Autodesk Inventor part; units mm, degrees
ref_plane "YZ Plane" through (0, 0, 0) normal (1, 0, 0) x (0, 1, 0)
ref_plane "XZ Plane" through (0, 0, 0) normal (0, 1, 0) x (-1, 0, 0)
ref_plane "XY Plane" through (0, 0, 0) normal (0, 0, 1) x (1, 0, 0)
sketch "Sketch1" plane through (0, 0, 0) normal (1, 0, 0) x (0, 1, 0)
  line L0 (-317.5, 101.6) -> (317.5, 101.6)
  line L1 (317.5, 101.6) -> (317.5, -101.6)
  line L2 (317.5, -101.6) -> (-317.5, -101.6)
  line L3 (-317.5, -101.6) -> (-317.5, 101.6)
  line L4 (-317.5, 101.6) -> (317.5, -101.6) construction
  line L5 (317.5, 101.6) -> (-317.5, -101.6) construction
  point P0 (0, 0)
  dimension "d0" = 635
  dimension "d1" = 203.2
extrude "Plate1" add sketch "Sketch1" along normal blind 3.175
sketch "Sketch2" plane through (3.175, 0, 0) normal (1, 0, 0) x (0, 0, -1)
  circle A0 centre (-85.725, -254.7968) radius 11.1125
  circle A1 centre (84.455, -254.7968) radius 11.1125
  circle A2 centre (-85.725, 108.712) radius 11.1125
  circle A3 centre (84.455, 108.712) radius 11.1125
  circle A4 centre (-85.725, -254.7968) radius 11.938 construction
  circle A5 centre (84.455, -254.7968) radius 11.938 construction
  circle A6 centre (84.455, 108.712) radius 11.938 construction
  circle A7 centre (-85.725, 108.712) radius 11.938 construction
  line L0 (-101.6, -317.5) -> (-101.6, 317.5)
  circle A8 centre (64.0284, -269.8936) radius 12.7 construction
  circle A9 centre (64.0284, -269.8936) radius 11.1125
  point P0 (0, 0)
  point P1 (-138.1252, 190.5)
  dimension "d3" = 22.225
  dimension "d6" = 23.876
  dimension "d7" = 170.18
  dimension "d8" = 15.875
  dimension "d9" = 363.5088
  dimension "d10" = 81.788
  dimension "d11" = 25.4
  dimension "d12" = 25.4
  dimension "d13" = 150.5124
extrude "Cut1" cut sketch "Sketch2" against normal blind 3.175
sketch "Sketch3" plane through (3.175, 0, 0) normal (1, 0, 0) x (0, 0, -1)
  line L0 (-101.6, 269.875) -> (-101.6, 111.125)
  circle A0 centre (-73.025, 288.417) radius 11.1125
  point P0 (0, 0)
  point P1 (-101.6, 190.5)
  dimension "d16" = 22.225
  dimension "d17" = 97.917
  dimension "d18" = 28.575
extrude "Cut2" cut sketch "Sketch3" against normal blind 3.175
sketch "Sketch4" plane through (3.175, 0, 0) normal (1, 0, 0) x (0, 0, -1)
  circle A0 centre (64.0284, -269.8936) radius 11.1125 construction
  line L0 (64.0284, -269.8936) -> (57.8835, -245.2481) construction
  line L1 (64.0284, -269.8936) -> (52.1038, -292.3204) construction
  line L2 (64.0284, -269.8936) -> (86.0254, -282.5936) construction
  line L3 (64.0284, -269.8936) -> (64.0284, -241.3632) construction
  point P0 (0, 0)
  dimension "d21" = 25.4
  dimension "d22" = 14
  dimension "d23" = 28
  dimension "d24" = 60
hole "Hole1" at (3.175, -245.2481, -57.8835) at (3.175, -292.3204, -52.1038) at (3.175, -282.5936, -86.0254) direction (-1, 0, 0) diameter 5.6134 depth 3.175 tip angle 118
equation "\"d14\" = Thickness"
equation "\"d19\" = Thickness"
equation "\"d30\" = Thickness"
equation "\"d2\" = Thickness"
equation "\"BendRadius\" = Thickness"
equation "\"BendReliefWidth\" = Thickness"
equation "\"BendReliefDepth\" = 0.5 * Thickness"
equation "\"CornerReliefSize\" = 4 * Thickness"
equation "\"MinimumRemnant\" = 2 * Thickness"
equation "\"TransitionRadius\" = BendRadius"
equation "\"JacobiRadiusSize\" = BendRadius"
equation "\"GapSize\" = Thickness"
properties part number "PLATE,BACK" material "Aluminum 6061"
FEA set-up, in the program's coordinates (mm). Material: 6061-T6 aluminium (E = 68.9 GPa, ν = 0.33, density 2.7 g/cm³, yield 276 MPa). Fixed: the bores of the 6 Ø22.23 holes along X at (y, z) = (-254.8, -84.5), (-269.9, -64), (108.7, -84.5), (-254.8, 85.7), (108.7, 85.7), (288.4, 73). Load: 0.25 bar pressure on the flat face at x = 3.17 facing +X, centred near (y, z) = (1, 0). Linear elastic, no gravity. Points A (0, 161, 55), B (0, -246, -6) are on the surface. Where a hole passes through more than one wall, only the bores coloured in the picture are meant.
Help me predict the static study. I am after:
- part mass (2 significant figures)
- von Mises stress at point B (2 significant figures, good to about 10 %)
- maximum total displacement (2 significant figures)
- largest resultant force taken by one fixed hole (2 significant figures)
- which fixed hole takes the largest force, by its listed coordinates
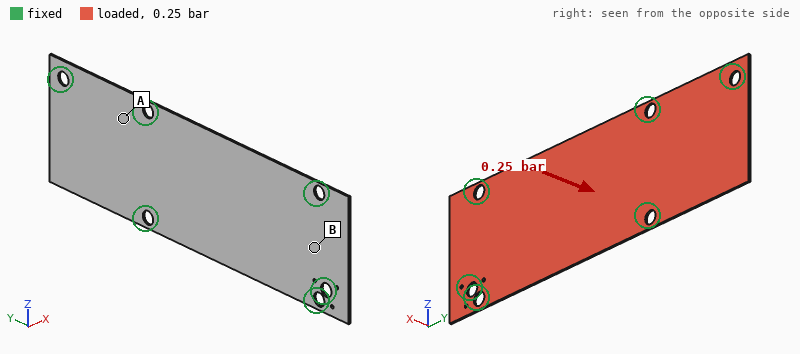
1.1 kg
60 MPa
6.0 mm
850 N
(108.7, -84.5)
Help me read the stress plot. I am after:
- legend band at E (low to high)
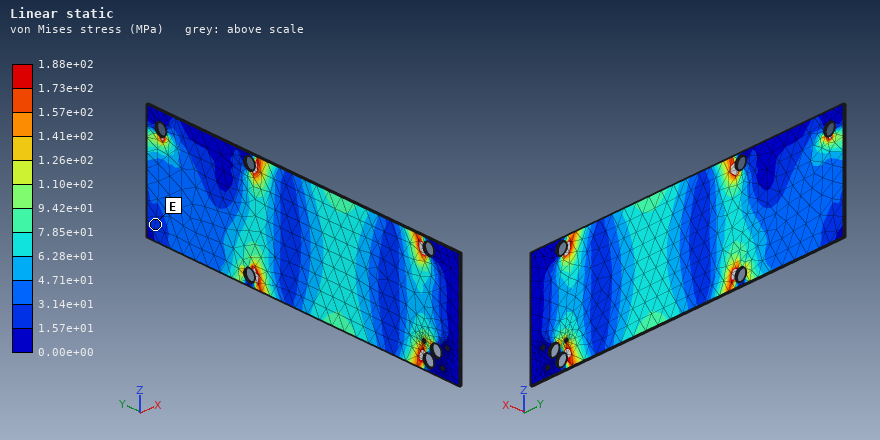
1.57e+01 to 3.14e+01 MPa
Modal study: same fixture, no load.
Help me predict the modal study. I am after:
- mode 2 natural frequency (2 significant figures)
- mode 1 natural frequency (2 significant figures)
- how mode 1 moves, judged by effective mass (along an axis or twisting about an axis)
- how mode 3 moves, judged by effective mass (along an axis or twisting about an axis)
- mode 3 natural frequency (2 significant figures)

160 Hz
130 Hz
along X
twisting about Y
210 Hz
